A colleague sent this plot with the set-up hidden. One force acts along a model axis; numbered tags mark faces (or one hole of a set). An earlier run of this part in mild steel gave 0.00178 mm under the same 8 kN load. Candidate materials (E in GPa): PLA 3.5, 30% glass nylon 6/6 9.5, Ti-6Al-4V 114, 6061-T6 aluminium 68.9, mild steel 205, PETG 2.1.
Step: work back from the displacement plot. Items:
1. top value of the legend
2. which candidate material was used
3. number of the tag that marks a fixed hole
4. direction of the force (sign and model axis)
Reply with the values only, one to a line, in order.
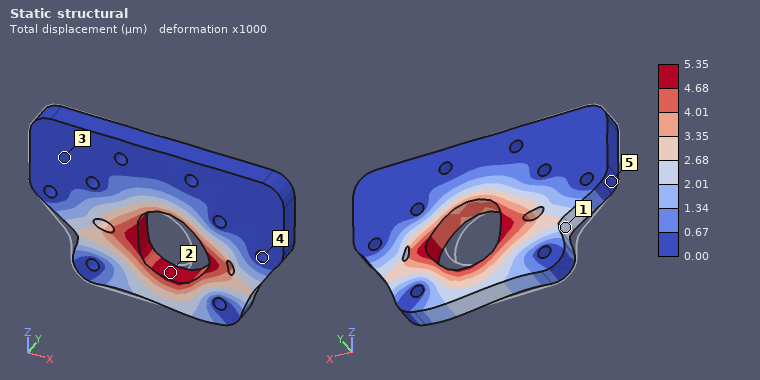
5.35 µm
6061-T6 aluminium
4
+X
